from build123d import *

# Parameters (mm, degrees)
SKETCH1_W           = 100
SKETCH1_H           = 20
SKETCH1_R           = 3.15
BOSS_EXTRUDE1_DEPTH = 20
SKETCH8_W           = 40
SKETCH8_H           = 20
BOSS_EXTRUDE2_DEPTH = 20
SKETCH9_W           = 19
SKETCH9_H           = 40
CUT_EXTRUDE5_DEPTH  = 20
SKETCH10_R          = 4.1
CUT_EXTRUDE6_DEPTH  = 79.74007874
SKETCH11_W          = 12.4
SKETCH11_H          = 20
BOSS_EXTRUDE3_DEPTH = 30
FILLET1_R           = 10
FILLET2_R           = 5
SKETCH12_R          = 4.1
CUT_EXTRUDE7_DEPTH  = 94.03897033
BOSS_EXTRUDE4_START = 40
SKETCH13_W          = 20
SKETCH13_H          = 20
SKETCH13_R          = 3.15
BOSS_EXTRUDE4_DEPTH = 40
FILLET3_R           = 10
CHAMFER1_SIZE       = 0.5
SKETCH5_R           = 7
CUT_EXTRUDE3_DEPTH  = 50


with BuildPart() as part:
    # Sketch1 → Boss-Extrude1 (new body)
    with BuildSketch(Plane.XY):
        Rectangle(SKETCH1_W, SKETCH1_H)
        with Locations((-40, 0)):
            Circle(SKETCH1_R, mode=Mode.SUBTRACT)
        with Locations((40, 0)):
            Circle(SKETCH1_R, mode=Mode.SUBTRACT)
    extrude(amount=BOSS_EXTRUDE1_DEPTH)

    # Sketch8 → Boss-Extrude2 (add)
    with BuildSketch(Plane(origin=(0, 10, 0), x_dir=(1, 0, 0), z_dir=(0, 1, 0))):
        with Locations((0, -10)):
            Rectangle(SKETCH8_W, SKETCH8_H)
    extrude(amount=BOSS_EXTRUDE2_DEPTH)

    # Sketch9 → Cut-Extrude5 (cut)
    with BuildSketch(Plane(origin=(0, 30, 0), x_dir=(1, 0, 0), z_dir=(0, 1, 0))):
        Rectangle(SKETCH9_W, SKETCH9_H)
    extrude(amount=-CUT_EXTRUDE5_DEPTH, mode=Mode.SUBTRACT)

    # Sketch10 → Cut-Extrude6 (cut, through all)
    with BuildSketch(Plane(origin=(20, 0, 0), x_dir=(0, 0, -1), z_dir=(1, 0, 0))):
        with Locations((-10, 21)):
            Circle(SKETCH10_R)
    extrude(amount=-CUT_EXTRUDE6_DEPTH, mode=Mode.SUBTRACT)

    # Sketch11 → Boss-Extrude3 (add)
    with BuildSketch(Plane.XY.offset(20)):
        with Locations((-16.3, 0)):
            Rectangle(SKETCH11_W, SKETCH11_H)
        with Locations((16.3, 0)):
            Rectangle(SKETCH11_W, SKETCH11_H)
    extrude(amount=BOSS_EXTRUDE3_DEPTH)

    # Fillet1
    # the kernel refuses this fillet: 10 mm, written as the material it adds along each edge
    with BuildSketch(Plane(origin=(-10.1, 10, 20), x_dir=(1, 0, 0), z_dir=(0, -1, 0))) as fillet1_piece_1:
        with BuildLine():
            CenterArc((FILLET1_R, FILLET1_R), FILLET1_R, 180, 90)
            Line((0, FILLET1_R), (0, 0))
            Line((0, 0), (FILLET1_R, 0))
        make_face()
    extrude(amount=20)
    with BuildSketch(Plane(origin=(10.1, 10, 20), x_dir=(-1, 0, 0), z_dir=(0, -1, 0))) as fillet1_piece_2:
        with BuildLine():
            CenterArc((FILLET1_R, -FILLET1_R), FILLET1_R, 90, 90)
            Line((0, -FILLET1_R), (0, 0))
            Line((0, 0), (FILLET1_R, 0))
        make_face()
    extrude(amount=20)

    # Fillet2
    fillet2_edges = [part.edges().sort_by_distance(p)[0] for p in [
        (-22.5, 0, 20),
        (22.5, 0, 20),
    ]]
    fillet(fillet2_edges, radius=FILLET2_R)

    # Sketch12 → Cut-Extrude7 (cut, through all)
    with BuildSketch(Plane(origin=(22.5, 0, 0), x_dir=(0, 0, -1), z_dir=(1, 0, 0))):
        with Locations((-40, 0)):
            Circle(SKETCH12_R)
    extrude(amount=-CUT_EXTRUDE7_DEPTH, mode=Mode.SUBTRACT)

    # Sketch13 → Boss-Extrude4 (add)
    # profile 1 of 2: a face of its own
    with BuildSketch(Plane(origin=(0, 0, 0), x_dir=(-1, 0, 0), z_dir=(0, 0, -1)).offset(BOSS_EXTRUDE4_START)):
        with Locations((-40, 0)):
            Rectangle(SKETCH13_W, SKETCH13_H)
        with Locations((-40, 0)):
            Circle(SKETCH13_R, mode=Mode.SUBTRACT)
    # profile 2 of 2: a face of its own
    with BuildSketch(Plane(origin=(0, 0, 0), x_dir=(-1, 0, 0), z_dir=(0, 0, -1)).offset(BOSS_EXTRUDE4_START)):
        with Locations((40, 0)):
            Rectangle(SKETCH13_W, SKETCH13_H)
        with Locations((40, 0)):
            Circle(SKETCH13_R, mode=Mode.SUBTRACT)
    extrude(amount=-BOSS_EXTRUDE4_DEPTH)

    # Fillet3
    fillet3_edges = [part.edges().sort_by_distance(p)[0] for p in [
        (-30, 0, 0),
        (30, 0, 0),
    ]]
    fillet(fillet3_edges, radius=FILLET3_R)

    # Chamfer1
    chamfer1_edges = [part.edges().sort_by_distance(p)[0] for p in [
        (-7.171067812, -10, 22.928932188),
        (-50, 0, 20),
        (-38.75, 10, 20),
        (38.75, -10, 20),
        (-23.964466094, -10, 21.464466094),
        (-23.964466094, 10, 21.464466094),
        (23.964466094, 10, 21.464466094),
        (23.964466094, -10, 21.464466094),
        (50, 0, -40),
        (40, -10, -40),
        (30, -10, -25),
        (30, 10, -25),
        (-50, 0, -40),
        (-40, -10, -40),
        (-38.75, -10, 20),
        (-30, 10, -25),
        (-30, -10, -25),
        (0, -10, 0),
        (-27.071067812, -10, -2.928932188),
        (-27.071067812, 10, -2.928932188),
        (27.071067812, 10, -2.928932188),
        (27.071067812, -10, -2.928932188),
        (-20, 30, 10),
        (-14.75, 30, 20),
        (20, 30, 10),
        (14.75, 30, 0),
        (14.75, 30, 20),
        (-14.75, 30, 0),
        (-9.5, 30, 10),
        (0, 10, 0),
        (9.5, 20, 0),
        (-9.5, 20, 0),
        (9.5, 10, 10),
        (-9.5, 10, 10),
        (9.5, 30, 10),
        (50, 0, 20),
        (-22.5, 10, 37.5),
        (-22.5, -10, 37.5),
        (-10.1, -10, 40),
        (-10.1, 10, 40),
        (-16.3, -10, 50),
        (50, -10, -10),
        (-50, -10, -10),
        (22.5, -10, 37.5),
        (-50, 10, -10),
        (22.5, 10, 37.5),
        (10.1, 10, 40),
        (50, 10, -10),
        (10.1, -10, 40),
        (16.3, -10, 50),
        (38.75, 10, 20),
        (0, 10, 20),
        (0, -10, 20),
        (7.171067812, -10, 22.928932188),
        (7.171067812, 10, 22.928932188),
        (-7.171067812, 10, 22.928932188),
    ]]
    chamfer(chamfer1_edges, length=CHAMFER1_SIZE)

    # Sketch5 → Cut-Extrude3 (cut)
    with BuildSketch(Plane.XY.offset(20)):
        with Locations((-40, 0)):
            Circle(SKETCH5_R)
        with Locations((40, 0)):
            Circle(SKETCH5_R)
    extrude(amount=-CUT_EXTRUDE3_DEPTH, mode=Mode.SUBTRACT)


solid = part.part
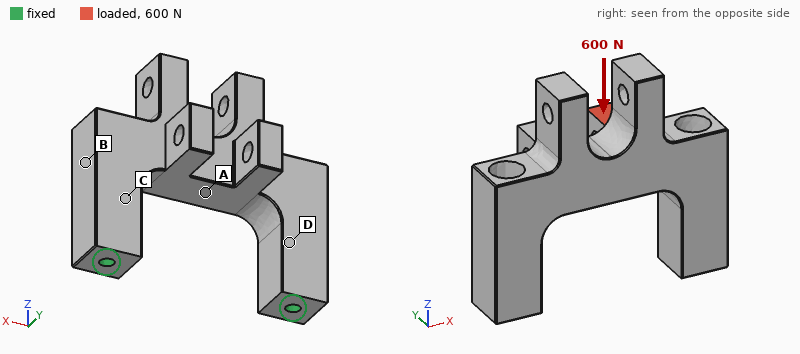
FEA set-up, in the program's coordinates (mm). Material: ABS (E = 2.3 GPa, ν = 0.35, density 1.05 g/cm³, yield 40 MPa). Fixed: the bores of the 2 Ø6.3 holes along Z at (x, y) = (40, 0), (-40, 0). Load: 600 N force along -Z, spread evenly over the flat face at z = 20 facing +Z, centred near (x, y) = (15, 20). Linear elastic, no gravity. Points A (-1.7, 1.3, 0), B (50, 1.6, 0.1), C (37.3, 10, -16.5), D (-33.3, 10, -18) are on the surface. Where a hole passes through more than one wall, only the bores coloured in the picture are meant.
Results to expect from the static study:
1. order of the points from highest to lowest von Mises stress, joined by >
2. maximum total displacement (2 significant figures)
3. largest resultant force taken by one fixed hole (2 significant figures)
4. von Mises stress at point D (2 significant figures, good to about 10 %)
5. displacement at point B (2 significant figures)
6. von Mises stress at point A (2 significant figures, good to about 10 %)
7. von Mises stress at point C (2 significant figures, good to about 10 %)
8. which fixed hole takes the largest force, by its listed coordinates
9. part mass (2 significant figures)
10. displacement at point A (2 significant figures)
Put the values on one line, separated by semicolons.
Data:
C > D > A > B; 1.3 mm; 430 N; 6.3 MPa; 0.31 mm; 4.7 MPa; 8.5 MPa; (40, 0); 83 g; 0.27 mm
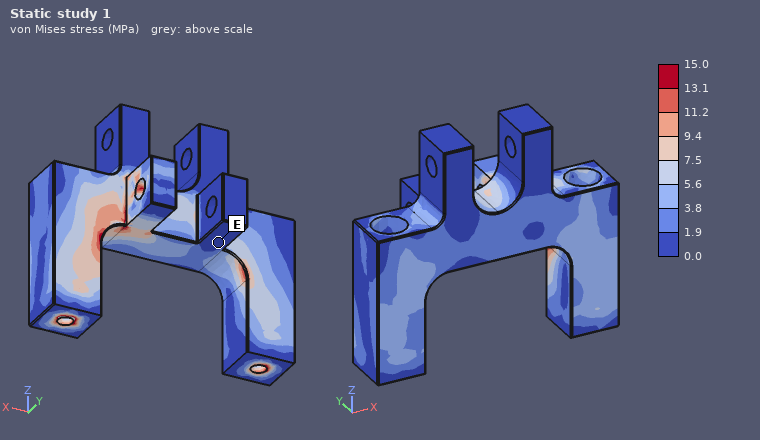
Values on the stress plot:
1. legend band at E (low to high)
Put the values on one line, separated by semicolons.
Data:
0.0 to 1.9 MPa
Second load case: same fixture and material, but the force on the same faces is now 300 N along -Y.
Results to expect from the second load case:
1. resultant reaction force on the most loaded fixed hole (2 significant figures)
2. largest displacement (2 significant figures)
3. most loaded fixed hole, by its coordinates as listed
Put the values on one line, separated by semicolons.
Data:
200 N; 1.3 mm; (40, 0)
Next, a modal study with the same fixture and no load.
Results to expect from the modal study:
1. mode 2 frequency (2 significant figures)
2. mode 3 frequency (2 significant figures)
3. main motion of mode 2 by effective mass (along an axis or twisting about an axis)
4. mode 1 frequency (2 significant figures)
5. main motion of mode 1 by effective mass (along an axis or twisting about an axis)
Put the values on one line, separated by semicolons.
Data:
950 Hz; 1200 Hz; along X; 430 Hz; along Y
